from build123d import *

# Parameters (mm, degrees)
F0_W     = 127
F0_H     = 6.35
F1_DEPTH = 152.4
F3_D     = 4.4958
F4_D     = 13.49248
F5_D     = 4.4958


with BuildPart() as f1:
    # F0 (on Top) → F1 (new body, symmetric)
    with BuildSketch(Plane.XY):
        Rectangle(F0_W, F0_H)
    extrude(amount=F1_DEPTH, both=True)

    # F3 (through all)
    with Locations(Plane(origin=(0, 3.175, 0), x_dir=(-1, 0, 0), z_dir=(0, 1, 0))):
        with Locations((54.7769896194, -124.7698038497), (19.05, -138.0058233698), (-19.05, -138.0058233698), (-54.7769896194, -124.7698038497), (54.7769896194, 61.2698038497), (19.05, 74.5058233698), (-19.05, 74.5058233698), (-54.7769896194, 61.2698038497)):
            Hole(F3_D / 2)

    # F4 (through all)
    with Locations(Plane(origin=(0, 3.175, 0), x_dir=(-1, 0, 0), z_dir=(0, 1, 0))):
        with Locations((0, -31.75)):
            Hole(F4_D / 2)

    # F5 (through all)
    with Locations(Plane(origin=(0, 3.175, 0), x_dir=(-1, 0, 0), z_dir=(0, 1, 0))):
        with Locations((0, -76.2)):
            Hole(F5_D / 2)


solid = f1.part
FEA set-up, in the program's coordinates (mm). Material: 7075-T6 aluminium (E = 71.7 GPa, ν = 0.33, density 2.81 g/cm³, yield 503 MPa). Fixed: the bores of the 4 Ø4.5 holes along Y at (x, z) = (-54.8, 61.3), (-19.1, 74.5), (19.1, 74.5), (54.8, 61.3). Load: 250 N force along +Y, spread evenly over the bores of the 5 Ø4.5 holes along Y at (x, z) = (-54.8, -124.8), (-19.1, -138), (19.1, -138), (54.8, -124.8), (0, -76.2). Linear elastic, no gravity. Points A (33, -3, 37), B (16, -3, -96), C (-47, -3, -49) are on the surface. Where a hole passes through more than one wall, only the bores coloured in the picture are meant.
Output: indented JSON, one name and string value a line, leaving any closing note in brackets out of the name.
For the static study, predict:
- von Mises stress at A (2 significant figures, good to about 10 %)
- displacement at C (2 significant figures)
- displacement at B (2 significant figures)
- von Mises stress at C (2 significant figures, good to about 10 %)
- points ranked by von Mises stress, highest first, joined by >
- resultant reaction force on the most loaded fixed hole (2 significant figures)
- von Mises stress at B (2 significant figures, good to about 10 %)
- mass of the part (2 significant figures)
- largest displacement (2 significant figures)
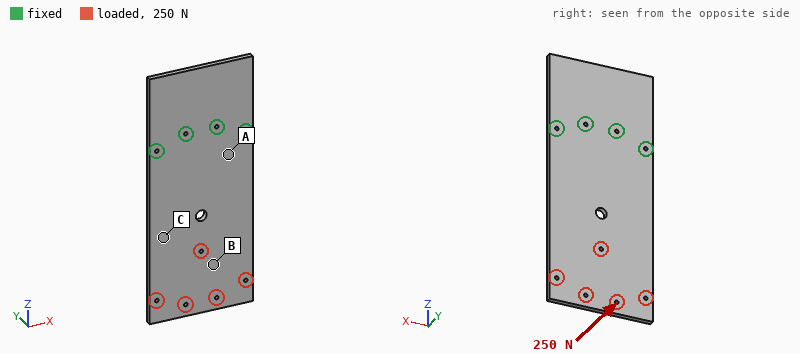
{
  "von Mises stress at A": "43 MPa",
  "displacement at C": "1.3 mm",
  "displacement at B": "2.3 mm",
  "von Mises stress at C": "22 MPa",
  "points ranked by von Mises stress, highest first, joined by >": "A > C > B",
  "resultant reaction force on the most loaded fixed hole": "220 N",
  "von Mises stress at B": "9.4 MPa",
  "mass of the part": "690 g",
  "largest displacement": "3.6 mm"
}
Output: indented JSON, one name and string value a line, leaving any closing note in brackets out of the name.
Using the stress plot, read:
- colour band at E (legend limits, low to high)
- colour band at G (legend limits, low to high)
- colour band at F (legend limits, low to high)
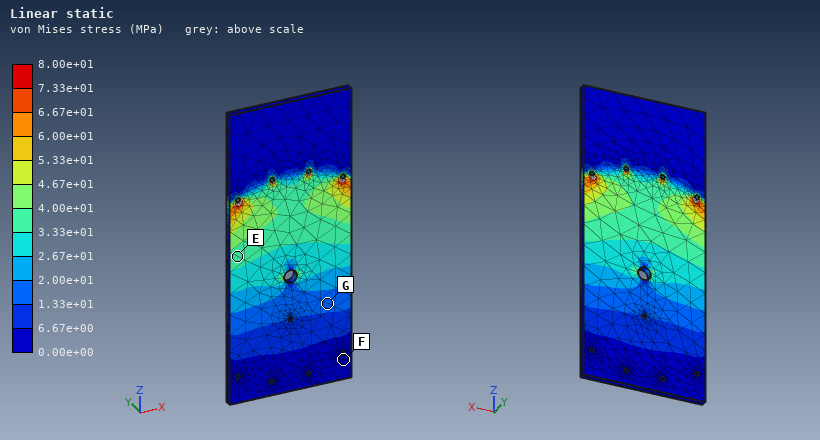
{
  "colour band at E": "3.33e+01 to 4.00e+01 MPa",
  "colour band at G": "1.33e+01 to 2.00e+01 MPa",
  "colour band at F": "0.00e+00 to 6.67e+00 MPa"
}
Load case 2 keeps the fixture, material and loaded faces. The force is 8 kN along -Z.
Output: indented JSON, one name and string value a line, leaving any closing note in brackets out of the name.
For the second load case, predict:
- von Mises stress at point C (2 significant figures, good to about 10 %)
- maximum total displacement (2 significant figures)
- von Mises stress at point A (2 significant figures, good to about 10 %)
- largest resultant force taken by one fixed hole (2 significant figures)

{
  "von Mises stress at point C": "9.5 MPa",
  "maximum total displacement": "30 µm",
  "von Mises stress at point A": "9.1 MPa",
  "largest resultant force taken by one fixed hole": "2.2 kN"
}
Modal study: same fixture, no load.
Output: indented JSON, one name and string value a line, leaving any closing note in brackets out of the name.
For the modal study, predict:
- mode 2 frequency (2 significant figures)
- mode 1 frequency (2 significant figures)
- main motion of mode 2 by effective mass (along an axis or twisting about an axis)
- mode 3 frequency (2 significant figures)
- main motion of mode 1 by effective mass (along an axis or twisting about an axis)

{
  "mode 2 frequency": "420 Hz",
  "mode 1 frequency": "110 Hz",
  "main motion of mode 2 by effective mass": "twisting about Z",
  "mode 3 frequency": "670 Hz",
  "main motion of mode 1 by effective mass": "along Y"
}
